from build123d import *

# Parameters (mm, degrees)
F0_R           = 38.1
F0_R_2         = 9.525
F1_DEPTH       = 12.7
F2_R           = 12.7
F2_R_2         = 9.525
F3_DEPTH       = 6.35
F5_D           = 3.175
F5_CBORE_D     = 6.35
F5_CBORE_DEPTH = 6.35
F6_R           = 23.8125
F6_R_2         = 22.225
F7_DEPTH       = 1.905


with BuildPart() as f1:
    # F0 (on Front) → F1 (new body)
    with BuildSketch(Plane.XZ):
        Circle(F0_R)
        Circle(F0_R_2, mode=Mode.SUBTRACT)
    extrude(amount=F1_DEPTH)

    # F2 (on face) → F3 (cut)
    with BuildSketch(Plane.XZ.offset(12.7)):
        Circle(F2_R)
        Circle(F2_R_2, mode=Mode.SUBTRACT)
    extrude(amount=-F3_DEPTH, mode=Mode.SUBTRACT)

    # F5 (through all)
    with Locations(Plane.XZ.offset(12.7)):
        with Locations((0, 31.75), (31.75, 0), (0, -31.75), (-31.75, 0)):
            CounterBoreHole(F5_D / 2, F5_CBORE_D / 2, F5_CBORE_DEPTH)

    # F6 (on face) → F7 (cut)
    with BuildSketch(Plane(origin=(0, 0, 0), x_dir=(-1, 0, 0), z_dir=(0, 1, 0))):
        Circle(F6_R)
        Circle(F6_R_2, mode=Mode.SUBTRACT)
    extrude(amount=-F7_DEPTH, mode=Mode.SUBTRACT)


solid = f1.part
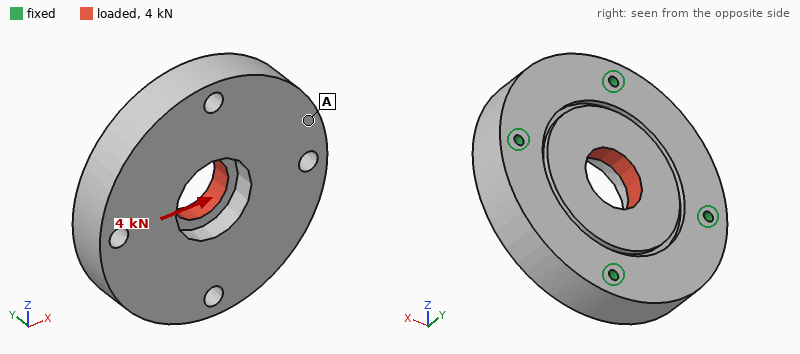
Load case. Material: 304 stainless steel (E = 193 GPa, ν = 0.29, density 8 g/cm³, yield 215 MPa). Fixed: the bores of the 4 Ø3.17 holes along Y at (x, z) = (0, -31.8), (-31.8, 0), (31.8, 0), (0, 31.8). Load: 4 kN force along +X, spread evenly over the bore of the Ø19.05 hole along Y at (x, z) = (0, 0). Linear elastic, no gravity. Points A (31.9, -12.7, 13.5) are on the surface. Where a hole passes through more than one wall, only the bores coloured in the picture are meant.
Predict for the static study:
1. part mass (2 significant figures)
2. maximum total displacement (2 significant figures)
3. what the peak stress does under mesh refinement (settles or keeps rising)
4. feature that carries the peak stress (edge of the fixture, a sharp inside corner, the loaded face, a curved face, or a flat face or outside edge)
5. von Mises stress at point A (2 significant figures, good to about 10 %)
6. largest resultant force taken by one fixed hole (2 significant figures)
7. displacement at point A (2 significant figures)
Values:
410 g
1.5 µm
keeps rising
edge of the fixture
2.4 MPa
1.1 kN
0.72 µm
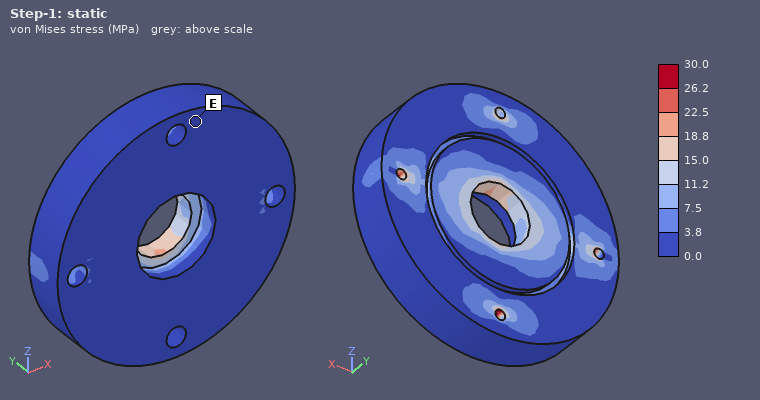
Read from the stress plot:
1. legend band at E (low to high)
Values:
0.0 to 3.8 MPa
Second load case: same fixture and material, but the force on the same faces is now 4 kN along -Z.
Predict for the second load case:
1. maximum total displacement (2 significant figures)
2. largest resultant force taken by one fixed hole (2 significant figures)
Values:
1.5 µm
1.1 kN
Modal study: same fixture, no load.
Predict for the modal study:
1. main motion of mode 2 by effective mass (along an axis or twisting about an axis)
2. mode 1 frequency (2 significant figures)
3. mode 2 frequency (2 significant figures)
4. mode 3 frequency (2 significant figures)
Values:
along Y
12 kHz
13 kHz
14 kHz
